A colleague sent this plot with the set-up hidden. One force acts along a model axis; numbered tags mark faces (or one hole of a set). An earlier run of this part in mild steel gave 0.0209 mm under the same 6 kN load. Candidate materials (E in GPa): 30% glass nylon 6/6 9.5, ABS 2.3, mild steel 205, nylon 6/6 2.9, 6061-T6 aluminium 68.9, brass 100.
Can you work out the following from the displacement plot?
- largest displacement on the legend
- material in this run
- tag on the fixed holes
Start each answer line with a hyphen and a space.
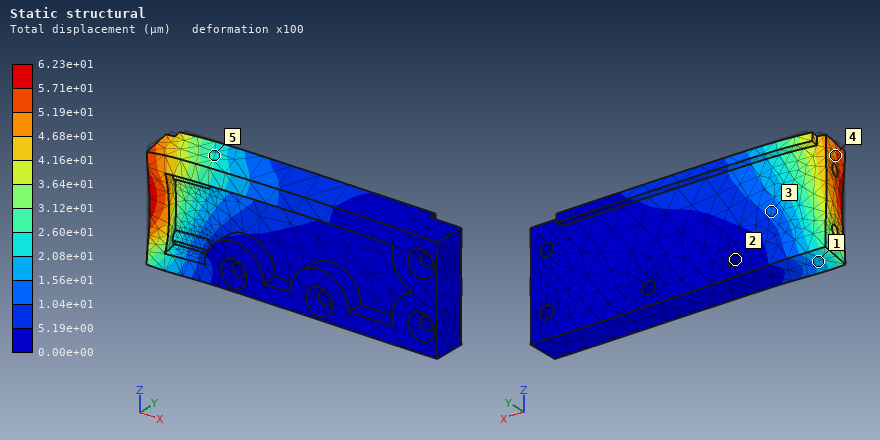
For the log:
- 6.23e+01 µm
- 6061-T6 aluminium
- 2
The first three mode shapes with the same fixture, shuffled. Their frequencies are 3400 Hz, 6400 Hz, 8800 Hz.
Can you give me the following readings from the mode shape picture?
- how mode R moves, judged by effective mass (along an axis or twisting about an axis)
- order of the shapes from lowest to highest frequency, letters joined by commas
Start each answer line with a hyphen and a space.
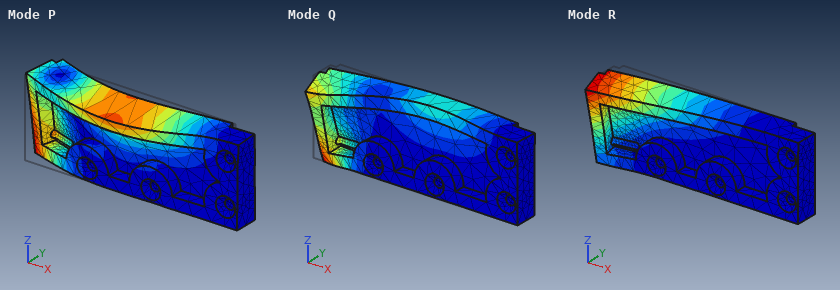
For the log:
- along Y
- R, P, Q
